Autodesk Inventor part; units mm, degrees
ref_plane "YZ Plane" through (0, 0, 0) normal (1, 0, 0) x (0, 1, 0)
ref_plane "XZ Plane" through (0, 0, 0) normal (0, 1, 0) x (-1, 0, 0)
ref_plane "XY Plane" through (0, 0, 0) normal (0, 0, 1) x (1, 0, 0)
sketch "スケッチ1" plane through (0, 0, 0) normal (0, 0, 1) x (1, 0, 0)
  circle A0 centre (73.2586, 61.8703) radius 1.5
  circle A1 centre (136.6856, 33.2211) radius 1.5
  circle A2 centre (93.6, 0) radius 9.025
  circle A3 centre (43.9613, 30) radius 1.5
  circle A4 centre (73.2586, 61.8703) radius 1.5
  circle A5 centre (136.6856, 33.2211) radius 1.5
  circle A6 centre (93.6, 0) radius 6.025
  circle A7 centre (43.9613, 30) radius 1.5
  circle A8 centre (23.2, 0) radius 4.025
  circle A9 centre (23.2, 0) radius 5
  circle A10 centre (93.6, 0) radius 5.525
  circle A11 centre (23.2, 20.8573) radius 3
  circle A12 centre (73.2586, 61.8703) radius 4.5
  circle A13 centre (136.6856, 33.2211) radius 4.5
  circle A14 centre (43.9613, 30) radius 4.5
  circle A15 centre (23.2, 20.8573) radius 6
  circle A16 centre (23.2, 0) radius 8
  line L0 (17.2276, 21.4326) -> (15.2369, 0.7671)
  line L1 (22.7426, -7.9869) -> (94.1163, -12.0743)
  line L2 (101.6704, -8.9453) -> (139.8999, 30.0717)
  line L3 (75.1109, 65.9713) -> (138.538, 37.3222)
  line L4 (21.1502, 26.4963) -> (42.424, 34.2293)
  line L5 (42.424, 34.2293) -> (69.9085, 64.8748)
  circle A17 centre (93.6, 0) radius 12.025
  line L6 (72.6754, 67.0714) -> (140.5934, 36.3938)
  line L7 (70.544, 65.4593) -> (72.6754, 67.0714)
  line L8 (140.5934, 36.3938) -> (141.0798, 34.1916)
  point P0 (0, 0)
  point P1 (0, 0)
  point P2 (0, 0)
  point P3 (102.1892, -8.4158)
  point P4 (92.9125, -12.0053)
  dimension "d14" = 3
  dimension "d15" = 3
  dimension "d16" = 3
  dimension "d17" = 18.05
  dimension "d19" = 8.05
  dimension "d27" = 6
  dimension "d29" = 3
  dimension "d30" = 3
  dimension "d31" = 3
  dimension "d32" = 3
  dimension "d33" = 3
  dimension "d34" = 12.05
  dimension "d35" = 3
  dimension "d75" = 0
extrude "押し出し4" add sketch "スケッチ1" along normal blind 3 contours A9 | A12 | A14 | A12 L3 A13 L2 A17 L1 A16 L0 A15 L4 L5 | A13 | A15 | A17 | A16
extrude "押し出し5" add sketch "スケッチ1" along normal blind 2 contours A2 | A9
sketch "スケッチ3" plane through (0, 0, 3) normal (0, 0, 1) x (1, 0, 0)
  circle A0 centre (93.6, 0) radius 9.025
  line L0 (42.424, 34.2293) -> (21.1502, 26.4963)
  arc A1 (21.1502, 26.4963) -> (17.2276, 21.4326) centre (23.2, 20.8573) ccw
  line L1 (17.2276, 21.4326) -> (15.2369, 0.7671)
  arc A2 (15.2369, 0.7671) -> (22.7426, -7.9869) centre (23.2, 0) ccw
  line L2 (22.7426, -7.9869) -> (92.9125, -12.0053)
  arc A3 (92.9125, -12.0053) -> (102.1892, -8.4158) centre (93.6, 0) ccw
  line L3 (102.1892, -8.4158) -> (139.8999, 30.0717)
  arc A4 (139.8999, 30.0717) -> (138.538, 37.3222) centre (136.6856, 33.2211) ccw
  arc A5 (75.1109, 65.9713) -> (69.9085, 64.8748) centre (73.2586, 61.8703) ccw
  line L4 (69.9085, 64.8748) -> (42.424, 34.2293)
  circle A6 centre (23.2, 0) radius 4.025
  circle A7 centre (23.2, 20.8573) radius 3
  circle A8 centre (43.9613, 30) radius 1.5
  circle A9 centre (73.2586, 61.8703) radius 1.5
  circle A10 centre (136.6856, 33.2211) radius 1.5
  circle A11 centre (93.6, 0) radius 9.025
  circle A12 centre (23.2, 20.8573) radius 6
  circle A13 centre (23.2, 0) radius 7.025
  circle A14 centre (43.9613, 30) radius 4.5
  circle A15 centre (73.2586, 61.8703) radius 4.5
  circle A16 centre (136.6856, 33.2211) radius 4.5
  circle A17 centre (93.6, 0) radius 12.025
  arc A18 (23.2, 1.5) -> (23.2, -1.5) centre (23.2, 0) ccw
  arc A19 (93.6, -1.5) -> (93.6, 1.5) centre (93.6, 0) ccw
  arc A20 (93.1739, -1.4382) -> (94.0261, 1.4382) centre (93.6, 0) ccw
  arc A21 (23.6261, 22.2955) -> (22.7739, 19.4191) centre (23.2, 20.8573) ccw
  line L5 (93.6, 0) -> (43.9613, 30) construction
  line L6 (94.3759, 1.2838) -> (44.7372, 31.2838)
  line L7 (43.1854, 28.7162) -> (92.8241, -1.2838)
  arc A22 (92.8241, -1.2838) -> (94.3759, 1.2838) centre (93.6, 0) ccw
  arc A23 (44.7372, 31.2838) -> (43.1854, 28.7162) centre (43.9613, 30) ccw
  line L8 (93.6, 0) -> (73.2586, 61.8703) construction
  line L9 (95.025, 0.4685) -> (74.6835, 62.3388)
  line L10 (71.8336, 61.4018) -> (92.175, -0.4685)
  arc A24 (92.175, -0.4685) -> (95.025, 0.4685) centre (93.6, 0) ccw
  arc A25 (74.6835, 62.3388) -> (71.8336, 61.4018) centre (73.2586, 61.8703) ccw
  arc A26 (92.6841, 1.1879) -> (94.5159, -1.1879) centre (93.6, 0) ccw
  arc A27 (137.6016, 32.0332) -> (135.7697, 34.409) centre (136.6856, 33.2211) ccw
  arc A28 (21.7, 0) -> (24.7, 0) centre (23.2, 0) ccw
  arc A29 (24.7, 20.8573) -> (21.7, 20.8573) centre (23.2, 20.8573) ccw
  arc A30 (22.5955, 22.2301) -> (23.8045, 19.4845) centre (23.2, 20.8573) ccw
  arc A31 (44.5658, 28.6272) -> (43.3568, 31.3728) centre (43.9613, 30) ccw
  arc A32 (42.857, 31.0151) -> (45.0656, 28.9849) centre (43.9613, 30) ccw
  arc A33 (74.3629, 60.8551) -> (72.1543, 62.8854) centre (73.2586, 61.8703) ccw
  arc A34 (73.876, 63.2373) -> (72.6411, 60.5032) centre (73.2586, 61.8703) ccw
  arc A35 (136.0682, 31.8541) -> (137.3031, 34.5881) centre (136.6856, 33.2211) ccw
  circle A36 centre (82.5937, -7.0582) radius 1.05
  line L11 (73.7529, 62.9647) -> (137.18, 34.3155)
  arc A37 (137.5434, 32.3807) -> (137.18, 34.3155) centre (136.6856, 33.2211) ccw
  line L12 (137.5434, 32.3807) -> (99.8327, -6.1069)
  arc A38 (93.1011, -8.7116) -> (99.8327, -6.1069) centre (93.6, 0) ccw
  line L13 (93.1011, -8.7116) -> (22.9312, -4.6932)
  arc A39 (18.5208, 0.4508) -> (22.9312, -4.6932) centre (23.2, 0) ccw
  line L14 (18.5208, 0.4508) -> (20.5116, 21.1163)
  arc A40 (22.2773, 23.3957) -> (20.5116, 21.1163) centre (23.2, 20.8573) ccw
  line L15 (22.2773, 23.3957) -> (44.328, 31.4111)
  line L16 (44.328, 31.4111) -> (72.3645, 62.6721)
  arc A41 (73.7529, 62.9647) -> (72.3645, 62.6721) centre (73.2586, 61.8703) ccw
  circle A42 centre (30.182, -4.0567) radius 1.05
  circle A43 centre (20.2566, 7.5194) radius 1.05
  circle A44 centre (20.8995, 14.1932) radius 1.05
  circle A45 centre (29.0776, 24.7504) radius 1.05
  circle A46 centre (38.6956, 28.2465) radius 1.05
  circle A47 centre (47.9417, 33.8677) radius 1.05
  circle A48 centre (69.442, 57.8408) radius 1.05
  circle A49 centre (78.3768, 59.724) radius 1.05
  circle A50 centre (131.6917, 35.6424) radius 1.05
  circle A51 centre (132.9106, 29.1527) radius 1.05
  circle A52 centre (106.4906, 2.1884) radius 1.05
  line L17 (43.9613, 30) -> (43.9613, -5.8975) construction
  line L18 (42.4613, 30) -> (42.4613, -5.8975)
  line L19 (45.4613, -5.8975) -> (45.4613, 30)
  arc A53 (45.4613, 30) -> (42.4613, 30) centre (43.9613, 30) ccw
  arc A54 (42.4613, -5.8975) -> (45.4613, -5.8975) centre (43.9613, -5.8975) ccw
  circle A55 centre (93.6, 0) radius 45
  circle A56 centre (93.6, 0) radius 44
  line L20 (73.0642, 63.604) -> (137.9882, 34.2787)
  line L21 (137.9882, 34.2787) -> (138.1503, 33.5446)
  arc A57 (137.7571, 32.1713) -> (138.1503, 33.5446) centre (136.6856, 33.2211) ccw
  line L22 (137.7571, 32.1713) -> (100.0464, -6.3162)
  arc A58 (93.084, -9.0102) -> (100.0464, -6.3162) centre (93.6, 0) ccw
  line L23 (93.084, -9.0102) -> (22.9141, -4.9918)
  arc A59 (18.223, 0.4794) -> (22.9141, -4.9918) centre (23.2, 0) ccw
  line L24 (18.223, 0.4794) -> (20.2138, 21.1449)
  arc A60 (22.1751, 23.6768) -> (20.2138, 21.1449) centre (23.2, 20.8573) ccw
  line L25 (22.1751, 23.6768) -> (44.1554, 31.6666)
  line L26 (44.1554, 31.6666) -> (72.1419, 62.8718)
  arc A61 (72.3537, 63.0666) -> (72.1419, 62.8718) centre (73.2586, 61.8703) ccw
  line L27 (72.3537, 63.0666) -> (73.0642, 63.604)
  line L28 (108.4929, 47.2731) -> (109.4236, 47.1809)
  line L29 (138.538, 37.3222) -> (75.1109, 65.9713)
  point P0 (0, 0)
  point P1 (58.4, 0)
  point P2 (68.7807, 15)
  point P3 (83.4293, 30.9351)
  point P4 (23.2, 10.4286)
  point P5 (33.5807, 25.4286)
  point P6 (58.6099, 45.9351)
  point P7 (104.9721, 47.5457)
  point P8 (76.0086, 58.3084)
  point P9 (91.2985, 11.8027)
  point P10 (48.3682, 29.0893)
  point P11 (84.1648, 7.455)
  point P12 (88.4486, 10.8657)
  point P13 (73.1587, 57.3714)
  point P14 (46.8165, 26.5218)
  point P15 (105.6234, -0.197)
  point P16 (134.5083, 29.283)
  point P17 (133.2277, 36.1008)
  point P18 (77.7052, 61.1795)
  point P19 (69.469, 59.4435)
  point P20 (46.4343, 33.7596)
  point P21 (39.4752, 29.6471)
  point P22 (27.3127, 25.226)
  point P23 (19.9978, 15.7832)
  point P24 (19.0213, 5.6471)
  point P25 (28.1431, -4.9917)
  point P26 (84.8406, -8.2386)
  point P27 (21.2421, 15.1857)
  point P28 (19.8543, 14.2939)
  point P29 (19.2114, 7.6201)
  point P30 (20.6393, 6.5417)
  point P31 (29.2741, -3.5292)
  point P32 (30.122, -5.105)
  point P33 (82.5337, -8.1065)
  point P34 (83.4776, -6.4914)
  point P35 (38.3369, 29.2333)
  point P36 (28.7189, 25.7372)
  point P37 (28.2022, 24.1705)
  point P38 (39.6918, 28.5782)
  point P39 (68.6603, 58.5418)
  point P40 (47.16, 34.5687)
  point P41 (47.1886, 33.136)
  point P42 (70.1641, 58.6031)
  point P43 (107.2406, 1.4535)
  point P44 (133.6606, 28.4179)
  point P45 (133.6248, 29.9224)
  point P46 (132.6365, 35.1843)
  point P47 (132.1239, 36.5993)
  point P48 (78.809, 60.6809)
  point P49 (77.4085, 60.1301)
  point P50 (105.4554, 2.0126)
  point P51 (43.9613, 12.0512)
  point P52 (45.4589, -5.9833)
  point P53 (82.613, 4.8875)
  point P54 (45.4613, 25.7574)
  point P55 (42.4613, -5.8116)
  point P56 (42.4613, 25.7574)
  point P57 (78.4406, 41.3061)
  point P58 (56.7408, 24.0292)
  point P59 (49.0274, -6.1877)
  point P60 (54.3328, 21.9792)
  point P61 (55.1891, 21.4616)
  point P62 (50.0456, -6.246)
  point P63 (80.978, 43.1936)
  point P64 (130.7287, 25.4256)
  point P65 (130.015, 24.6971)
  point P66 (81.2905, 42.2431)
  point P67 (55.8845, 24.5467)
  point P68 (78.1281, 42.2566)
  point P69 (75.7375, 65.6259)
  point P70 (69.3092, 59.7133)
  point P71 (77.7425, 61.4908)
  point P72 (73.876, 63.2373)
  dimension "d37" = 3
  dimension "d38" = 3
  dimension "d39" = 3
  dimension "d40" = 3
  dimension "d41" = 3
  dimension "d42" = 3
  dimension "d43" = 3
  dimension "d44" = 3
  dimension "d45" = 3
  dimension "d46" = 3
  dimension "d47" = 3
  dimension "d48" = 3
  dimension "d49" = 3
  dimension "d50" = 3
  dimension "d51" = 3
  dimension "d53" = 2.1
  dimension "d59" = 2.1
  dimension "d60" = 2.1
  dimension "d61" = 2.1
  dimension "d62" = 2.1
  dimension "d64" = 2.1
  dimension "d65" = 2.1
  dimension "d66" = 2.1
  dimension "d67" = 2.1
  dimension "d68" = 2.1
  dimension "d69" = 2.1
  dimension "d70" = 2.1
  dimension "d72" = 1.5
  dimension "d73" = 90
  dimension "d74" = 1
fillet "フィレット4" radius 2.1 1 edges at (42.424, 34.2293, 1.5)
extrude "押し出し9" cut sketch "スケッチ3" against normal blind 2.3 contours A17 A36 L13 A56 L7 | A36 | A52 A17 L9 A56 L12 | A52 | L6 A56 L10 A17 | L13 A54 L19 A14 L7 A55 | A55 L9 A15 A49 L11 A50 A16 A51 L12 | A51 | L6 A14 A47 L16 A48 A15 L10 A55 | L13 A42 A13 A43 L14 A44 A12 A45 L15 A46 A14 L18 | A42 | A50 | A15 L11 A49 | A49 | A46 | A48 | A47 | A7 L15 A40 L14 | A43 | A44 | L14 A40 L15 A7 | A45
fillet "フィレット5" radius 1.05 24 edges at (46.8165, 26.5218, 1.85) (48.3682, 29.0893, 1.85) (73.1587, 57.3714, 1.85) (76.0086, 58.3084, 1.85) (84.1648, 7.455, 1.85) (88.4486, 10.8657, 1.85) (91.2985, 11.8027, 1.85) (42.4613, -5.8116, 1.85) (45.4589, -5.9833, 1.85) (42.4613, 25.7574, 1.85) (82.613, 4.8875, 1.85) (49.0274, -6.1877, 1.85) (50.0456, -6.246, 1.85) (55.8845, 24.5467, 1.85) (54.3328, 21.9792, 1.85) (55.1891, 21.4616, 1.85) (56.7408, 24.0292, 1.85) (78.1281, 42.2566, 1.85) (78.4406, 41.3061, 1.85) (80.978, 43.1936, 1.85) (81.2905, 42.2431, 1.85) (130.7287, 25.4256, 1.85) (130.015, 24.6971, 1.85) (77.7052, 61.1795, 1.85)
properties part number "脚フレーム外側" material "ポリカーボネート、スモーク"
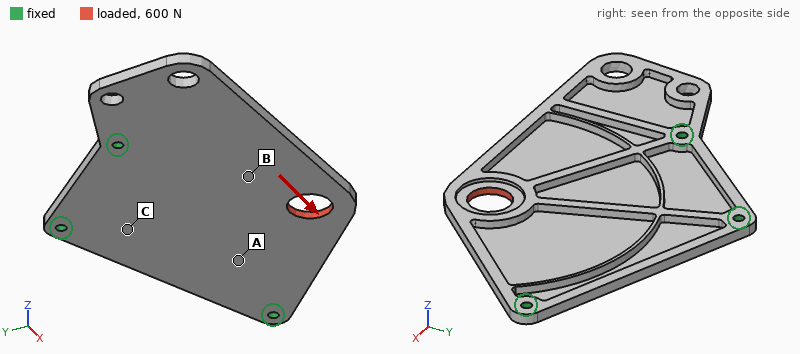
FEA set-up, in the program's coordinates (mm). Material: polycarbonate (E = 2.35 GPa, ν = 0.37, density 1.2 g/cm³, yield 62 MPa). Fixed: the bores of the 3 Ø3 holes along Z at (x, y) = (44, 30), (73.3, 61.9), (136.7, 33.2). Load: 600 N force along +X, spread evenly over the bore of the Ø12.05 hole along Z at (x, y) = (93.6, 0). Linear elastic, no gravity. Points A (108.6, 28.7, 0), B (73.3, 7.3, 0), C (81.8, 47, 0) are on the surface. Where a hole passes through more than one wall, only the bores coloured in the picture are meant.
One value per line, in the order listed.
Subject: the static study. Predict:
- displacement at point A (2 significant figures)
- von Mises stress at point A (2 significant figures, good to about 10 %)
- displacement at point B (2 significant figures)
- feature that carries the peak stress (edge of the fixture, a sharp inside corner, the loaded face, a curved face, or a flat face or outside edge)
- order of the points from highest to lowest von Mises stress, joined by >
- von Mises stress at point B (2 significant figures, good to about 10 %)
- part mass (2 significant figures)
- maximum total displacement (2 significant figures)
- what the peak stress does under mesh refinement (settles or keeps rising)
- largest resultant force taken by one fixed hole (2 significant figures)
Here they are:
0.35 mm
7.4 MPa
0.29 mm
edge of the fixture
B > A > C
12 MPa
10 g
1.1 mm
keeps rising
370 N
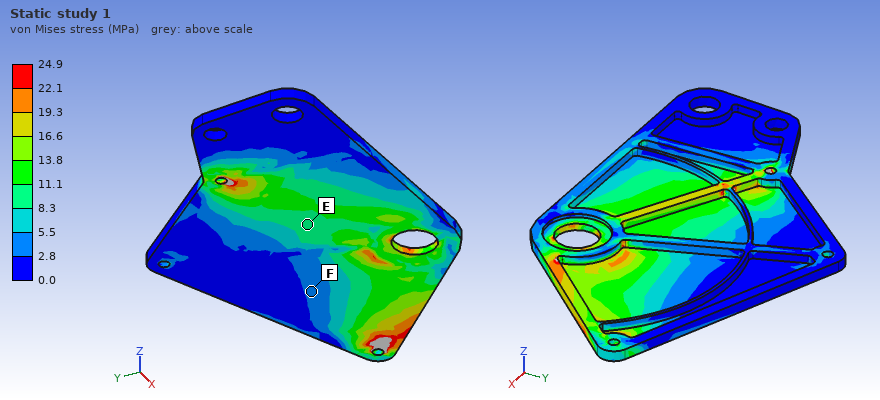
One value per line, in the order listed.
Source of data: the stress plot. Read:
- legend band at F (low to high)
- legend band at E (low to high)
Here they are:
2.8 to 5.5 MPa
8.3 to 11.1 MPa
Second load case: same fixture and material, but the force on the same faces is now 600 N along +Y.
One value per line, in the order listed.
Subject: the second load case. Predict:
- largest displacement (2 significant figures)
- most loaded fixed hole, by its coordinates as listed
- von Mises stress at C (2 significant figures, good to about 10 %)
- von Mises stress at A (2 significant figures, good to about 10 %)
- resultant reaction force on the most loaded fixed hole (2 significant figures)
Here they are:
1.4 mm
(73.3, 61.9)
13 MPa
4.8 MPa
290 N
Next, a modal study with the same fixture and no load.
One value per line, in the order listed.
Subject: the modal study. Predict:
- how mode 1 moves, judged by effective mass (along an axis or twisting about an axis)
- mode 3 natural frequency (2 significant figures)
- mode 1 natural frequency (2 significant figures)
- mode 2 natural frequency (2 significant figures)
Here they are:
along Z
580 Hz
210 Hz
290 Hz
